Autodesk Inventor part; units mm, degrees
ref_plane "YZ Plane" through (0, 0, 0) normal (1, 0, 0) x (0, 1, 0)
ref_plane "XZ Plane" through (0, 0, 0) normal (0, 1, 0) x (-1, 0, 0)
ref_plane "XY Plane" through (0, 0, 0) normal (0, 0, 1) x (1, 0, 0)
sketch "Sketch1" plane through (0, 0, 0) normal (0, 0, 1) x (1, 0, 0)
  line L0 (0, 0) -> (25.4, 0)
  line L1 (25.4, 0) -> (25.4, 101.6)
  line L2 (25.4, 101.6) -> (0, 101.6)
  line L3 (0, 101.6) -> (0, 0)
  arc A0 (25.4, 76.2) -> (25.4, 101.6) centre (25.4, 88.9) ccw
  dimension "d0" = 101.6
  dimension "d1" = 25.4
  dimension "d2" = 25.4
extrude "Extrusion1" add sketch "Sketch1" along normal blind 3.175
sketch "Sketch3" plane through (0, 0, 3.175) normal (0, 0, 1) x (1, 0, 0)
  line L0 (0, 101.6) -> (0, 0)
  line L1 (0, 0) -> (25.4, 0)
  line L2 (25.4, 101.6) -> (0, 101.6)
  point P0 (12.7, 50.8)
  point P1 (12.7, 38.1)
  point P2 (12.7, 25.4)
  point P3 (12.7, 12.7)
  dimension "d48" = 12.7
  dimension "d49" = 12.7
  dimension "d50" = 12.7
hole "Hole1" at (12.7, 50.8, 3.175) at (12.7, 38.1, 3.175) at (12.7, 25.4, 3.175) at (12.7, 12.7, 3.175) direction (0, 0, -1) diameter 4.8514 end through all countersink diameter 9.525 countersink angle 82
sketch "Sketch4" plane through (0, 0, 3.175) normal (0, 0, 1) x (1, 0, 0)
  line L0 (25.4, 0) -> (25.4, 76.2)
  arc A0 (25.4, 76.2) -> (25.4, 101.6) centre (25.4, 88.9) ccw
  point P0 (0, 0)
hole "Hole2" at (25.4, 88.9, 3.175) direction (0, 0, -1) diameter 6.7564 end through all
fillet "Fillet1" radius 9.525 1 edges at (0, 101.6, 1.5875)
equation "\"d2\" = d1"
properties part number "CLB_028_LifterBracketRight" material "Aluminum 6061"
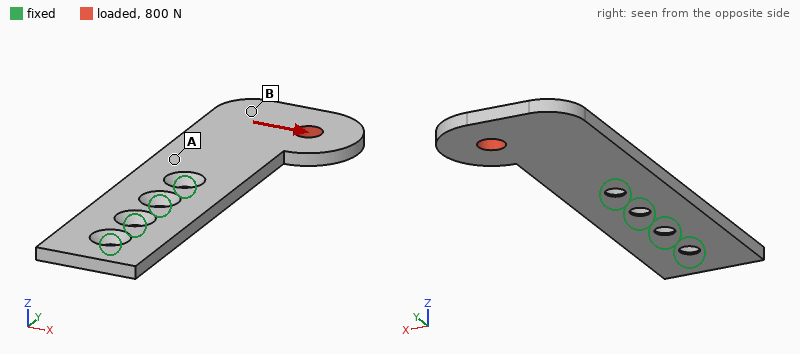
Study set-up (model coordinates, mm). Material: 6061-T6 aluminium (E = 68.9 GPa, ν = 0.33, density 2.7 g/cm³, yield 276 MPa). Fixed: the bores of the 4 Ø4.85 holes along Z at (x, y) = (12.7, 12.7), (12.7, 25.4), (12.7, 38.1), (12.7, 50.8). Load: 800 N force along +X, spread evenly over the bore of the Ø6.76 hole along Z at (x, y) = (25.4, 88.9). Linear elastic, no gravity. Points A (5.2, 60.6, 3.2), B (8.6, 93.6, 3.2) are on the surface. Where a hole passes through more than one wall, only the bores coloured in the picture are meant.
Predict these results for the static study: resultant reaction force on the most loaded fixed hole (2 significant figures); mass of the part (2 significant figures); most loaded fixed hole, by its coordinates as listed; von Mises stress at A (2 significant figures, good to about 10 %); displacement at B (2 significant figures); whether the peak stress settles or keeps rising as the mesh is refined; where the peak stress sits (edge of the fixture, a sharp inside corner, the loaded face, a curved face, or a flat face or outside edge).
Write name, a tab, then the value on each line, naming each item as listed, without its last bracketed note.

resultant reaction force on the most loaded fixed hole	1.8 kN
mass of the part	23 g
most loaded fixed hole, by its coordinates as listed	(12.7, 50.8)
von Mises stress at A	48 MPa
displacement at B	0.16 mm
whether the peak stress settles or keeps rising as the mesh is refined	keeps rising
where the peak stress sits	edge of the fixture
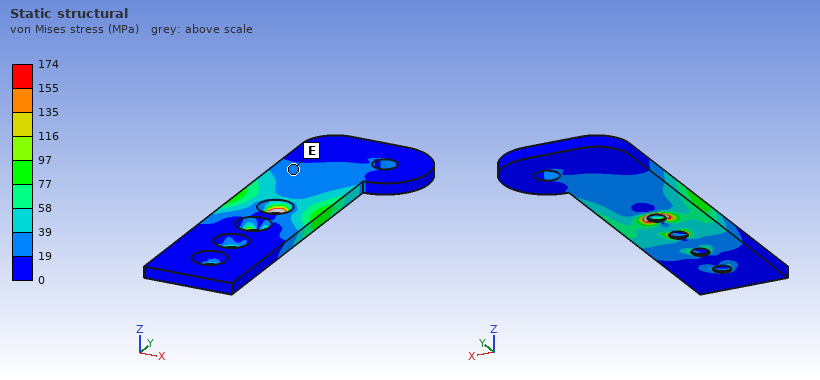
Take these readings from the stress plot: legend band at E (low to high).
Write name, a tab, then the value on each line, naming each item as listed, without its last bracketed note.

legend band at E	19 to 39 MPa
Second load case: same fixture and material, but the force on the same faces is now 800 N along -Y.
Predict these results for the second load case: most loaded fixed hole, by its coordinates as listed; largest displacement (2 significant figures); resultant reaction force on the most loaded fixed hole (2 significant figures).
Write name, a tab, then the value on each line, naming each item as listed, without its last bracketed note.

most loaded fixed hole, by its coordinates as listed	(12.7, 50.8)
largest displacement	86 µm
resultant reaction force on the most loaded fixed hole	550 N
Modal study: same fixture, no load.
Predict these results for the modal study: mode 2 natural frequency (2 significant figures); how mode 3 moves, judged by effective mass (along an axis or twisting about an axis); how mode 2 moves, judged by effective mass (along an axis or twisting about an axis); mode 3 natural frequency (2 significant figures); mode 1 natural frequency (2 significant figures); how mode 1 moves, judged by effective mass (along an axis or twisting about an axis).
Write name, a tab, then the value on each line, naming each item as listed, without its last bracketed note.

mode 2 natural frequency	2100 Hz
how mode 3 moves, judged by effective mass	along X
how mode 2 moves, judged by effective mass	twisting about Y
mode 3 natural frequency	4100 Hz
mode 1 natural frequency	780 Hz
how mode 1 moves, judged by effective mass	along Z
